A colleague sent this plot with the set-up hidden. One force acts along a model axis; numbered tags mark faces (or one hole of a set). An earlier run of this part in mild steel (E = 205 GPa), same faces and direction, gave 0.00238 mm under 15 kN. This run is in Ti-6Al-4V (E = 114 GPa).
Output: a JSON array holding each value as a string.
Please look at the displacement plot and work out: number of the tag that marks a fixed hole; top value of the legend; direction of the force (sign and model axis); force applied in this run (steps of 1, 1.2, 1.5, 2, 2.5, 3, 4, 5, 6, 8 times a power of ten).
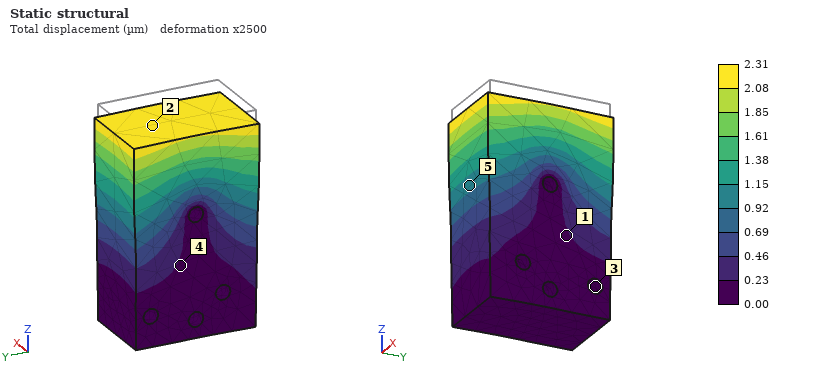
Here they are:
["3", "2.31 µm", "-Z", "8 kN"]
